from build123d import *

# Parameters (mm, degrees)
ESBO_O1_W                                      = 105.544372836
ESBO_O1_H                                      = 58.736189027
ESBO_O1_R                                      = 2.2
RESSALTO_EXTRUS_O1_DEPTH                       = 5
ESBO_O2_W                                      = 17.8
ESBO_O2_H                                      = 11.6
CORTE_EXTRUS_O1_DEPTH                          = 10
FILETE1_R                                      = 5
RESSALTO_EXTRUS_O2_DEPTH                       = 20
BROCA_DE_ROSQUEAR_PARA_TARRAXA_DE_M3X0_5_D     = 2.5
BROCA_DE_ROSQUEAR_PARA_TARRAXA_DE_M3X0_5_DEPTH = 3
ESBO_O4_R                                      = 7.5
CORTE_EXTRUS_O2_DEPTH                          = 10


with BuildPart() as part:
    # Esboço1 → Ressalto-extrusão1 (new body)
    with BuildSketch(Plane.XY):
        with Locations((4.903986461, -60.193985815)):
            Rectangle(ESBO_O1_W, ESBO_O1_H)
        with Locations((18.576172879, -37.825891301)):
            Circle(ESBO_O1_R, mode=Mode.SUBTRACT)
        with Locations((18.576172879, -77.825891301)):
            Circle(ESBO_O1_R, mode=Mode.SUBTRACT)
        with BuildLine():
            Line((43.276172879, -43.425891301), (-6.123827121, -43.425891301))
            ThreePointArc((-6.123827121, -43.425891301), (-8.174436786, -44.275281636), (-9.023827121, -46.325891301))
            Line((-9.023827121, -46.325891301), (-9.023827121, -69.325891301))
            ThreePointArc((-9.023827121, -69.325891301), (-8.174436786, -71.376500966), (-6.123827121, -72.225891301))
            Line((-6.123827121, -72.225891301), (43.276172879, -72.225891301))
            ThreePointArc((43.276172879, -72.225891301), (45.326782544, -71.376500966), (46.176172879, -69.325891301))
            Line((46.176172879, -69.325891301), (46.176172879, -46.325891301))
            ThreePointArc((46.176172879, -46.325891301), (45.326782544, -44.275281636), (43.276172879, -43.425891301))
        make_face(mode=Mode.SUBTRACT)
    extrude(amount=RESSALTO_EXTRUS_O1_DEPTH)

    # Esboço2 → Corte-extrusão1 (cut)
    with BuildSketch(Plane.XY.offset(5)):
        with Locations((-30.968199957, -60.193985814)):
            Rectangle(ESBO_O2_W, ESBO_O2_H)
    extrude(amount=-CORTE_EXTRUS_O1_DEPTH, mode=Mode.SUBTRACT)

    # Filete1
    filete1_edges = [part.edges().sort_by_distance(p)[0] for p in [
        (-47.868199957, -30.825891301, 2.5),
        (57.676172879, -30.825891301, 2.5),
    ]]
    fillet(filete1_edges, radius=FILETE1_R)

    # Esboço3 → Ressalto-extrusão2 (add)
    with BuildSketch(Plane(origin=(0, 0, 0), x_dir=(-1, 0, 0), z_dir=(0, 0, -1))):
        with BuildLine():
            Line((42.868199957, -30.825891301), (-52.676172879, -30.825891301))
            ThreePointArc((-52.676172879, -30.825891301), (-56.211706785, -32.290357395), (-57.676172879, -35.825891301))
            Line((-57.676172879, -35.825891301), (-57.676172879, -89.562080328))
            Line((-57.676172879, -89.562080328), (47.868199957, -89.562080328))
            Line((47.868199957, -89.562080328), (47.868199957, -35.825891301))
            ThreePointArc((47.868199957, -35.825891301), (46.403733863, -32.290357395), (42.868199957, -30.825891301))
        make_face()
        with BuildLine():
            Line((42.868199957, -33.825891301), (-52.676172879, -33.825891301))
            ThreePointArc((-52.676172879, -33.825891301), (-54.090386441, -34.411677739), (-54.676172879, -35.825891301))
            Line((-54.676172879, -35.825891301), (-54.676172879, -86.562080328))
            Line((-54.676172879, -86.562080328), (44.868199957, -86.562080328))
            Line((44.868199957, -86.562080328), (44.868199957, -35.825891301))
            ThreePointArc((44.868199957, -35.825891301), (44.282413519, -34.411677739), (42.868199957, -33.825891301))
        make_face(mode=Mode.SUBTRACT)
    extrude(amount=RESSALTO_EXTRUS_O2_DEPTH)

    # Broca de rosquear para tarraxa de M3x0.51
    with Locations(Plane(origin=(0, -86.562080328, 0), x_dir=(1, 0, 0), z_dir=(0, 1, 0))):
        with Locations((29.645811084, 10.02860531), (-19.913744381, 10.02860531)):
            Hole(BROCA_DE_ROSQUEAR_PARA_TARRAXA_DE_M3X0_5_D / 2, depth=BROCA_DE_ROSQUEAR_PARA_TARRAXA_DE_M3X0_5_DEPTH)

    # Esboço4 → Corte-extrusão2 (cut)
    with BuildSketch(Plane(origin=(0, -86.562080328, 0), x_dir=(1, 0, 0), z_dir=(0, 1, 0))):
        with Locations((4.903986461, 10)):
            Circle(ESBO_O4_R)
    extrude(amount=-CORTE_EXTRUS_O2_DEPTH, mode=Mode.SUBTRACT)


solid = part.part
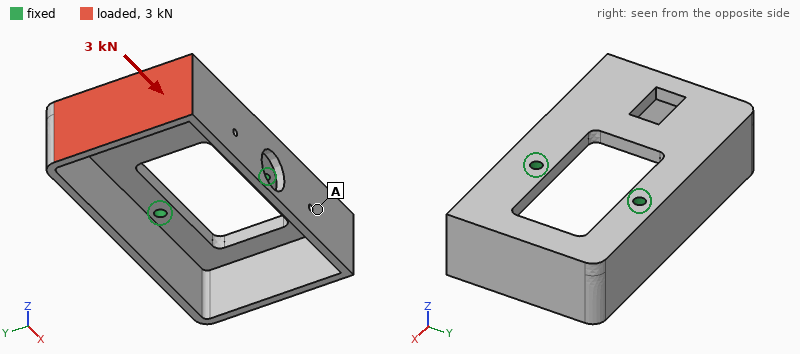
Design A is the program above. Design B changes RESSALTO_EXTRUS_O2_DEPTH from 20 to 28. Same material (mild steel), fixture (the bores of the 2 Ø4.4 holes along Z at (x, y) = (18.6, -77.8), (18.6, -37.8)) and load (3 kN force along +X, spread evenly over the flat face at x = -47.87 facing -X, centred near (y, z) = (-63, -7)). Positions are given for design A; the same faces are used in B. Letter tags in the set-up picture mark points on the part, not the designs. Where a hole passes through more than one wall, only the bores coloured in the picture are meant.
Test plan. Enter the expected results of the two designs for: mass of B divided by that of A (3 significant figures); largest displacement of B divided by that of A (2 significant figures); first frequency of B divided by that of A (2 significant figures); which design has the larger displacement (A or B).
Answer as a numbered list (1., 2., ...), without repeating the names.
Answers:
1. 1.19
2. 1.3
3. 0.91
4. B
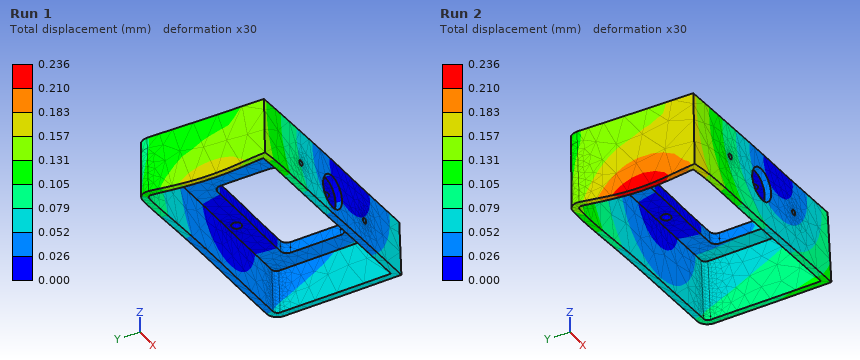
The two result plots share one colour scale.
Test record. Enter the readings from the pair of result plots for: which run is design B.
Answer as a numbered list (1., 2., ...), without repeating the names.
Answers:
1. Run 2
